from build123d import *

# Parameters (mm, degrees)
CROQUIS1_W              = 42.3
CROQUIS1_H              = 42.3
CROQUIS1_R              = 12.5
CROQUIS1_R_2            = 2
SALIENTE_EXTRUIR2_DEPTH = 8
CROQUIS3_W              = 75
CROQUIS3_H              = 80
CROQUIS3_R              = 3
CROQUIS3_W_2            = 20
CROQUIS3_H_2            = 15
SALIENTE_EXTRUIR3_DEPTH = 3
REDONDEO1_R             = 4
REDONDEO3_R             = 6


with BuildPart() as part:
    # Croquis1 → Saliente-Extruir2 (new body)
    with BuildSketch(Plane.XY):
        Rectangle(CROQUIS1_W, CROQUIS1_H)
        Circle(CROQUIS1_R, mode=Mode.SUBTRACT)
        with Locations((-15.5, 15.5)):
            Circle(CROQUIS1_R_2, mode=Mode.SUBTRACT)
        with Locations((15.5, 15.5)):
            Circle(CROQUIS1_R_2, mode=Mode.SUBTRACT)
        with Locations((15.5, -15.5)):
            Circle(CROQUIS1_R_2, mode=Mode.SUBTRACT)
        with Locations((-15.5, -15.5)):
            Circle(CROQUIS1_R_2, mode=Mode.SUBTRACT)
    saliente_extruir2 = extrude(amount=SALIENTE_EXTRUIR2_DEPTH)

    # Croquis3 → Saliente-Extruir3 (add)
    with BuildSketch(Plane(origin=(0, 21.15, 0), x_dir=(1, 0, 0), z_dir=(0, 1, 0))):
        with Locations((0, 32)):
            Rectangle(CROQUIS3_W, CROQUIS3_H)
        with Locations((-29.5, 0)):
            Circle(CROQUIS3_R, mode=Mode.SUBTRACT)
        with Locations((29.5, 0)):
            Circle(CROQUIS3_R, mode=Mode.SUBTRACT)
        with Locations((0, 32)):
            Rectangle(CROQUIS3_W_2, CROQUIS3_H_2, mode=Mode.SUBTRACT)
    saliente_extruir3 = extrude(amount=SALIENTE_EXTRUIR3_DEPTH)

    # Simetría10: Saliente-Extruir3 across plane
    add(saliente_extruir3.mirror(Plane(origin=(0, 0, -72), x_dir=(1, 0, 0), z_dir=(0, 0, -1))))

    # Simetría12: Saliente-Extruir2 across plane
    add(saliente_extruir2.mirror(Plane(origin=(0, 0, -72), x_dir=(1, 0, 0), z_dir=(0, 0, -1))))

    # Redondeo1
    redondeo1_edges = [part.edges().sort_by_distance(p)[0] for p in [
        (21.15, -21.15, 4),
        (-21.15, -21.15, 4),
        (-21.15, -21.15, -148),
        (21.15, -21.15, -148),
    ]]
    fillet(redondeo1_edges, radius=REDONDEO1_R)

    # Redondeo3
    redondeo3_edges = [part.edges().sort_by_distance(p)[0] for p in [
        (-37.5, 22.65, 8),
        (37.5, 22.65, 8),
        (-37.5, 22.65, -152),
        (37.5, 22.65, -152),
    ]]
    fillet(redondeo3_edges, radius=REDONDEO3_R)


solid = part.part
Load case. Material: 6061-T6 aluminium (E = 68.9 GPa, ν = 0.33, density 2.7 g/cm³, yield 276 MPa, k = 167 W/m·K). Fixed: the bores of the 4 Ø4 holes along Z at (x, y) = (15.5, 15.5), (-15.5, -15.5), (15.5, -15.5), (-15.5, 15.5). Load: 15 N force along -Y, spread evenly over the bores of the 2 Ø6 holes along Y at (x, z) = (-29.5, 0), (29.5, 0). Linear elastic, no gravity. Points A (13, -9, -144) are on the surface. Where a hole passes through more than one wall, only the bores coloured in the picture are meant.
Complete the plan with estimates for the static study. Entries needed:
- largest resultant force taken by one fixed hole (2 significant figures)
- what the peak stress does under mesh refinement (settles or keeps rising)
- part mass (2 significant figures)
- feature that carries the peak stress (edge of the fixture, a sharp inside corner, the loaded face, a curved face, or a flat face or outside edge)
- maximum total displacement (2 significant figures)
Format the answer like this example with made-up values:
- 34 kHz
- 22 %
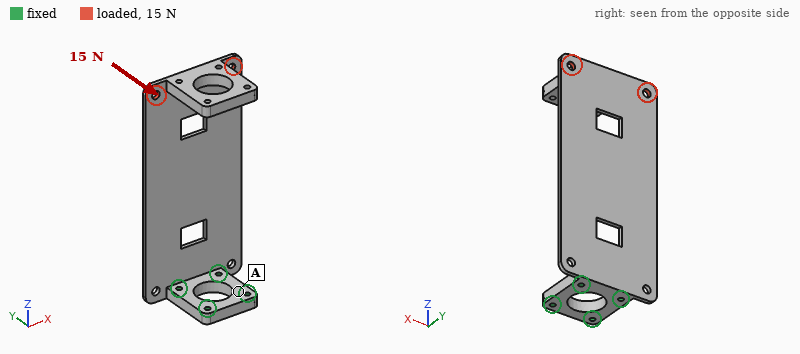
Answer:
- 27 N
- keeps rising
- 140 g
- a sharp inside corner
- 1.8 mm
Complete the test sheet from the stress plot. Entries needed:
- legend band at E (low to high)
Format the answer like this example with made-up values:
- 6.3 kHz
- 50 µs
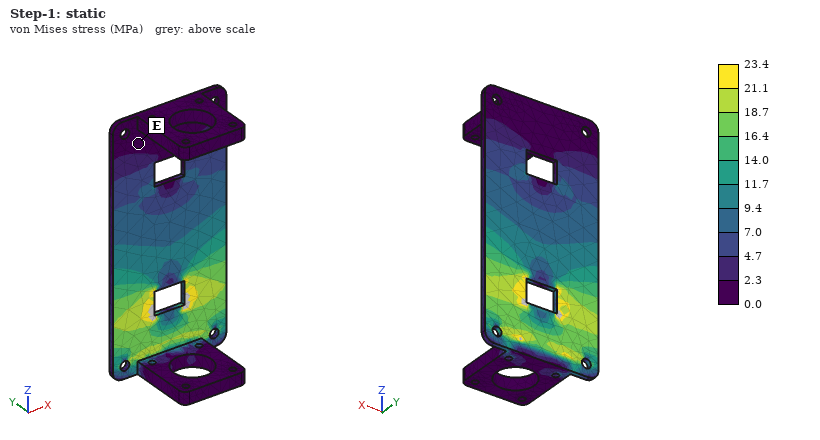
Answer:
- 0.0 to 2.3 MPa
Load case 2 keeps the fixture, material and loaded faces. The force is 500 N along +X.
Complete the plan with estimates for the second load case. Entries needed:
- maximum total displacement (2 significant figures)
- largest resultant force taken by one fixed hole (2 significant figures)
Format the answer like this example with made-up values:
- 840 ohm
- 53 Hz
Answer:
- 0.34 mm
- 2.2 kN
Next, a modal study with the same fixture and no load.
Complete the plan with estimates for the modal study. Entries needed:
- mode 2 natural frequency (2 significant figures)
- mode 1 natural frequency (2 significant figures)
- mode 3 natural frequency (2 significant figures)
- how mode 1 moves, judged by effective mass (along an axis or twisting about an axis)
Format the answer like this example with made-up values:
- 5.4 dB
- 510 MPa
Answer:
- 280 Hz
- 67 Hz
- 410 Hz
- along Y
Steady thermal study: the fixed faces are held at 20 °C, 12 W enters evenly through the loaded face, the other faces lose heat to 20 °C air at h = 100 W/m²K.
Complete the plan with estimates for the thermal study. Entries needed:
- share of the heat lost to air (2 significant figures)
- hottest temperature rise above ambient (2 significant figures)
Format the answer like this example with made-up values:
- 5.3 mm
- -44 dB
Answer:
- 95 %
- 15 K
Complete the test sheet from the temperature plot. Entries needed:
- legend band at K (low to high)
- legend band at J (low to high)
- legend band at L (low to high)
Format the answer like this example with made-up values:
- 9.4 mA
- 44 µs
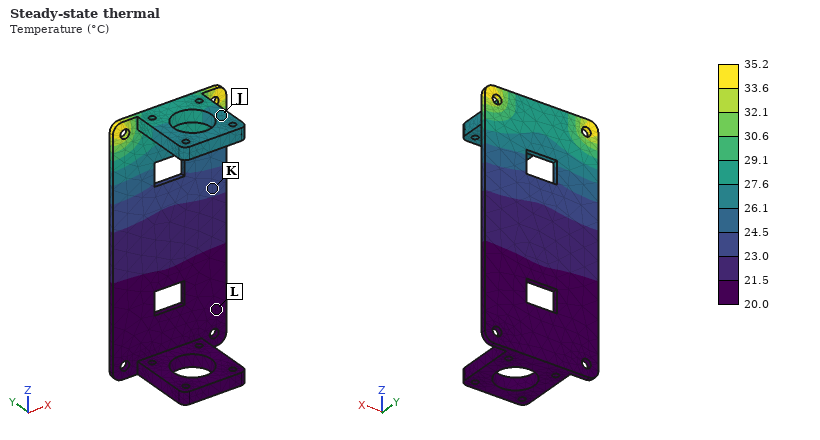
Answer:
- 23.0 to 24.5 °C
- 26.1 to 27.6 °C
- 20.0 to 21.5 °C
